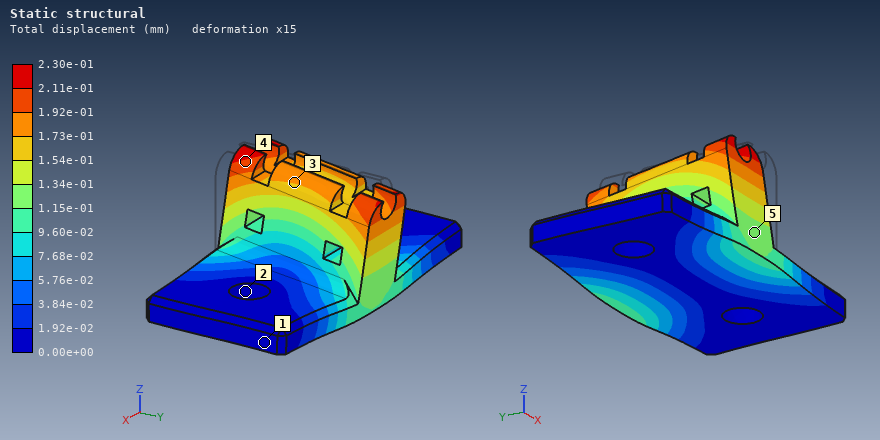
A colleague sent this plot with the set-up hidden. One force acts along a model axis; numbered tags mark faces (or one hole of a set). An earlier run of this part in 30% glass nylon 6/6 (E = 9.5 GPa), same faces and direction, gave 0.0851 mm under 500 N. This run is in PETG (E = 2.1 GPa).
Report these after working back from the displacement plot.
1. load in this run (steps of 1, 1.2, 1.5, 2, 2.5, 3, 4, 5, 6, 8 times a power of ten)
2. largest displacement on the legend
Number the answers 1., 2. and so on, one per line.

1. 300 N
2. 2.30e-01 mm
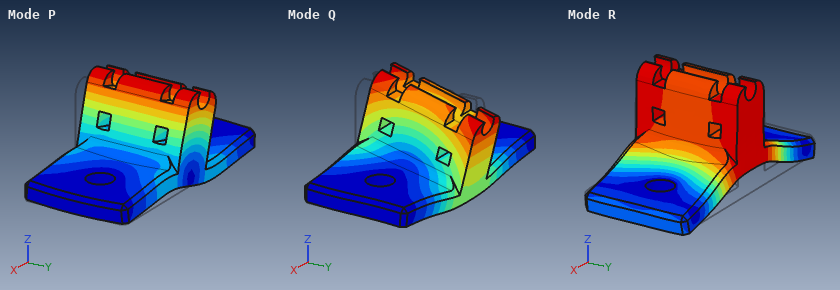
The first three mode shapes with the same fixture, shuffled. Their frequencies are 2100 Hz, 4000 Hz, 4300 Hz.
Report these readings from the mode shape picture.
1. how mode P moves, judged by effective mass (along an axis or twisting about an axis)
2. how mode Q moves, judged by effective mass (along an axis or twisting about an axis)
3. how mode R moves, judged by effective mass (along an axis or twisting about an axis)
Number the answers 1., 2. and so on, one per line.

1. along X
2. along Y
3. along Z
